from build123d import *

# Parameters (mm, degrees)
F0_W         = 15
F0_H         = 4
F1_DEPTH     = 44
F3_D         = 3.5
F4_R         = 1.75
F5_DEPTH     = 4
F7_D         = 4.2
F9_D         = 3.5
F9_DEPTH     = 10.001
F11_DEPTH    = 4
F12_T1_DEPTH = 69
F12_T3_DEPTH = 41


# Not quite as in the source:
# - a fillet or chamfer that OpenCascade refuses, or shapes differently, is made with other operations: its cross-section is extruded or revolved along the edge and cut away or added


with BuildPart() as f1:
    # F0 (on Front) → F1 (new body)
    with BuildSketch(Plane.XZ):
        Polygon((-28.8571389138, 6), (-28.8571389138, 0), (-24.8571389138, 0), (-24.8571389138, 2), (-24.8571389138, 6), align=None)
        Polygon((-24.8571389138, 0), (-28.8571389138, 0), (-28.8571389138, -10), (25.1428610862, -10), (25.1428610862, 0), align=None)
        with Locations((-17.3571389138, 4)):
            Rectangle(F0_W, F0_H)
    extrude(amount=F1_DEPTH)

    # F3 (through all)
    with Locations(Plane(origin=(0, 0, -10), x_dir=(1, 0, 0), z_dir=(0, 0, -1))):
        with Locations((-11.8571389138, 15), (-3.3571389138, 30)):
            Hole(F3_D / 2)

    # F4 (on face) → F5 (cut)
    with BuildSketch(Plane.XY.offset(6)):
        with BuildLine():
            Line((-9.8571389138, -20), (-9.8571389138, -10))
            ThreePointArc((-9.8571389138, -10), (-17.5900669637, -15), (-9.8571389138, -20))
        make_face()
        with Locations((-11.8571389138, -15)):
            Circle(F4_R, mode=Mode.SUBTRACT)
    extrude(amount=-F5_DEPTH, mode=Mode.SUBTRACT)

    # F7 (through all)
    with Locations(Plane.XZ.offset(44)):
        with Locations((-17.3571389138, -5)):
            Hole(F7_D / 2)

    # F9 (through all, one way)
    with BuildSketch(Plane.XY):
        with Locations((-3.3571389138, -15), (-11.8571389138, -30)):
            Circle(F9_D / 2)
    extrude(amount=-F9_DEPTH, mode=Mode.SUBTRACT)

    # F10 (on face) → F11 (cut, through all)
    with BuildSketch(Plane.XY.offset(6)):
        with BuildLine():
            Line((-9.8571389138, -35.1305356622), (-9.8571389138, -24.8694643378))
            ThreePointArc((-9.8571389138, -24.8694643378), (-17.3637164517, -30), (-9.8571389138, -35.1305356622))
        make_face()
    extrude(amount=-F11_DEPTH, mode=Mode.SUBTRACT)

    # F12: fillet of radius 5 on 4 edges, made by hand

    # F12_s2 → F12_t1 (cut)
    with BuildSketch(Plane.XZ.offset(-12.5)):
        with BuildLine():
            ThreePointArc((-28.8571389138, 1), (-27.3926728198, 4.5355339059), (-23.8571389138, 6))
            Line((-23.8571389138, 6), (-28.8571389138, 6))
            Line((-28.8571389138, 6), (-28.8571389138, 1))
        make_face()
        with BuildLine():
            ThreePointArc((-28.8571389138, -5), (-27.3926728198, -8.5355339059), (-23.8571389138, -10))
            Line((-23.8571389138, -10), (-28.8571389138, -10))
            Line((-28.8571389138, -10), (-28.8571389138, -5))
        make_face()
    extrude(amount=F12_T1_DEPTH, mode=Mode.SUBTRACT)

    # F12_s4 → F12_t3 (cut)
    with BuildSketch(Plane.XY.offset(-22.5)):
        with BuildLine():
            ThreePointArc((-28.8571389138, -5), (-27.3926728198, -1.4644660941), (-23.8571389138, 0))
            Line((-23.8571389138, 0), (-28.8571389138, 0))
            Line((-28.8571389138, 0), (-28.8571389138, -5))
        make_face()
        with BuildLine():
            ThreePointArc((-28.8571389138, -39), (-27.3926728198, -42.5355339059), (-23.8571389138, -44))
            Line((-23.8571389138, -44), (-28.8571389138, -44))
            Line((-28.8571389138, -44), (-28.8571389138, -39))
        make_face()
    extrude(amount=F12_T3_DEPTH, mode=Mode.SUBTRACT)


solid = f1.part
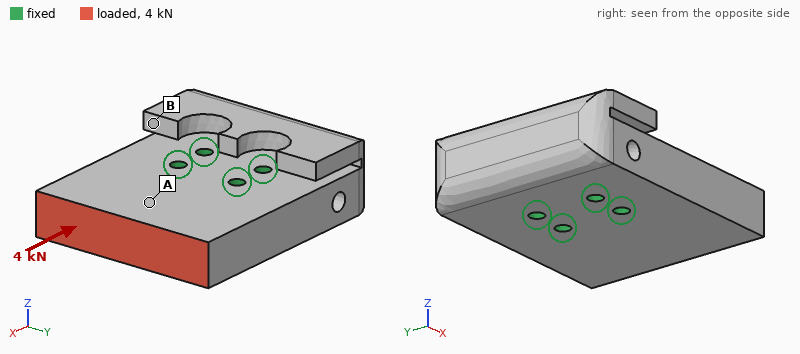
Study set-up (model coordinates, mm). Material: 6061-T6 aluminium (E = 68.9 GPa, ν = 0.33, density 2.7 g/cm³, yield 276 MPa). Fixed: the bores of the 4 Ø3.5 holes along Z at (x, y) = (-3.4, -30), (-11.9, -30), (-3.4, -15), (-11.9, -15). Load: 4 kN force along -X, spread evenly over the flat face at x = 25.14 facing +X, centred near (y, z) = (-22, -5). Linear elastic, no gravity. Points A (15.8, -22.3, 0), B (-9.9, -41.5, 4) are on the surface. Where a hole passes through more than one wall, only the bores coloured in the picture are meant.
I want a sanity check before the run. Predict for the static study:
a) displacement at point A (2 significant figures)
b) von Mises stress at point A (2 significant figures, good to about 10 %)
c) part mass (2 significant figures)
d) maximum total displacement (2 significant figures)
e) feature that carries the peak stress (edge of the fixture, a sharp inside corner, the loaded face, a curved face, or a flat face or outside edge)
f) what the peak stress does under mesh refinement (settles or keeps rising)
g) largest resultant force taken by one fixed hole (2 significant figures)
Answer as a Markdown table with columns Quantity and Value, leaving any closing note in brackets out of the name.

| Quantity | Value |
|---|---|
| displacement at point A | 3.0 µm |
| von Mises stress at point A | 10 MPa |
| part mass | 68 g |
| maximum total displacement | 5.3 µm |
| feature that carries the peak stress | edge of the fixture |
| what the peak stress does under mesh refinement | keeps rising |
| largest resultant force taken by one fixed hole | 1.5 kN |
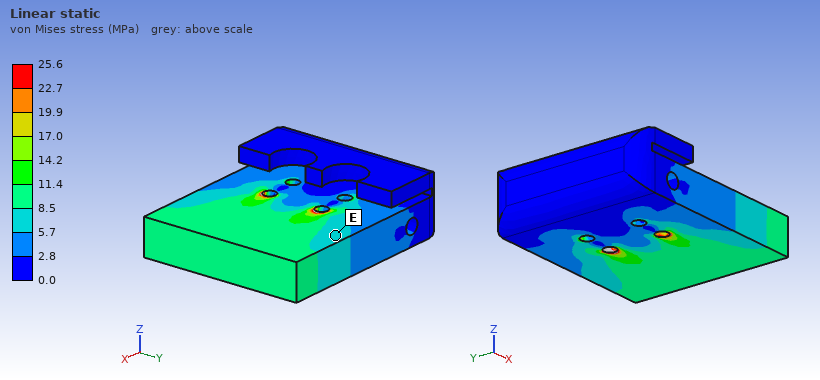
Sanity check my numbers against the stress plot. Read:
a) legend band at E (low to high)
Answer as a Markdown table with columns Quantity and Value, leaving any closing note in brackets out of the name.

| Quantity | Value |
|---|---|
| legend band at E | 5.7 to 8.5 MPa |
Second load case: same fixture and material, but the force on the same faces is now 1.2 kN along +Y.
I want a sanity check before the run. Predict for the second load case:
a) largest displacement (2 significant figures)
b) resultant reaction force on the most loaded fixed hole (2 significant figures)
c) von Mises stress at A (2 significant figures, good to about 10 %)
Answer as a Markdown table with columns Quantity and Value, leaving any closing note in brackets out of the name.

| Quantity | Value |
|---|---|
| largest displacement | 11 µm |
| resultant reaction force on the most loaded fixed hole | 1.4 kN |
| von Mises stress at A | 8.2 MPa |
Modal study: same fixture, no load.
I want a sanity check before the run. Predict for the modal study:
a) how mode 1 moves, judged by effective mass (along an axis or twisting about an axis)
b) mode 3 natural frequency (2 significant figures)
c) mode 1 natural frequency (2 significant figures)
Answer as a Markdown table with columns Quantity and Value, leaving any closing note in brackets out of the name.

| Quantity | Value |
|---|---|
| how mode 1 moves, judged by effective mass | along Z |
| mode 3 natural frequency | 9800 Hz |
| mode 1 natural frequency | 8400 Hz |
